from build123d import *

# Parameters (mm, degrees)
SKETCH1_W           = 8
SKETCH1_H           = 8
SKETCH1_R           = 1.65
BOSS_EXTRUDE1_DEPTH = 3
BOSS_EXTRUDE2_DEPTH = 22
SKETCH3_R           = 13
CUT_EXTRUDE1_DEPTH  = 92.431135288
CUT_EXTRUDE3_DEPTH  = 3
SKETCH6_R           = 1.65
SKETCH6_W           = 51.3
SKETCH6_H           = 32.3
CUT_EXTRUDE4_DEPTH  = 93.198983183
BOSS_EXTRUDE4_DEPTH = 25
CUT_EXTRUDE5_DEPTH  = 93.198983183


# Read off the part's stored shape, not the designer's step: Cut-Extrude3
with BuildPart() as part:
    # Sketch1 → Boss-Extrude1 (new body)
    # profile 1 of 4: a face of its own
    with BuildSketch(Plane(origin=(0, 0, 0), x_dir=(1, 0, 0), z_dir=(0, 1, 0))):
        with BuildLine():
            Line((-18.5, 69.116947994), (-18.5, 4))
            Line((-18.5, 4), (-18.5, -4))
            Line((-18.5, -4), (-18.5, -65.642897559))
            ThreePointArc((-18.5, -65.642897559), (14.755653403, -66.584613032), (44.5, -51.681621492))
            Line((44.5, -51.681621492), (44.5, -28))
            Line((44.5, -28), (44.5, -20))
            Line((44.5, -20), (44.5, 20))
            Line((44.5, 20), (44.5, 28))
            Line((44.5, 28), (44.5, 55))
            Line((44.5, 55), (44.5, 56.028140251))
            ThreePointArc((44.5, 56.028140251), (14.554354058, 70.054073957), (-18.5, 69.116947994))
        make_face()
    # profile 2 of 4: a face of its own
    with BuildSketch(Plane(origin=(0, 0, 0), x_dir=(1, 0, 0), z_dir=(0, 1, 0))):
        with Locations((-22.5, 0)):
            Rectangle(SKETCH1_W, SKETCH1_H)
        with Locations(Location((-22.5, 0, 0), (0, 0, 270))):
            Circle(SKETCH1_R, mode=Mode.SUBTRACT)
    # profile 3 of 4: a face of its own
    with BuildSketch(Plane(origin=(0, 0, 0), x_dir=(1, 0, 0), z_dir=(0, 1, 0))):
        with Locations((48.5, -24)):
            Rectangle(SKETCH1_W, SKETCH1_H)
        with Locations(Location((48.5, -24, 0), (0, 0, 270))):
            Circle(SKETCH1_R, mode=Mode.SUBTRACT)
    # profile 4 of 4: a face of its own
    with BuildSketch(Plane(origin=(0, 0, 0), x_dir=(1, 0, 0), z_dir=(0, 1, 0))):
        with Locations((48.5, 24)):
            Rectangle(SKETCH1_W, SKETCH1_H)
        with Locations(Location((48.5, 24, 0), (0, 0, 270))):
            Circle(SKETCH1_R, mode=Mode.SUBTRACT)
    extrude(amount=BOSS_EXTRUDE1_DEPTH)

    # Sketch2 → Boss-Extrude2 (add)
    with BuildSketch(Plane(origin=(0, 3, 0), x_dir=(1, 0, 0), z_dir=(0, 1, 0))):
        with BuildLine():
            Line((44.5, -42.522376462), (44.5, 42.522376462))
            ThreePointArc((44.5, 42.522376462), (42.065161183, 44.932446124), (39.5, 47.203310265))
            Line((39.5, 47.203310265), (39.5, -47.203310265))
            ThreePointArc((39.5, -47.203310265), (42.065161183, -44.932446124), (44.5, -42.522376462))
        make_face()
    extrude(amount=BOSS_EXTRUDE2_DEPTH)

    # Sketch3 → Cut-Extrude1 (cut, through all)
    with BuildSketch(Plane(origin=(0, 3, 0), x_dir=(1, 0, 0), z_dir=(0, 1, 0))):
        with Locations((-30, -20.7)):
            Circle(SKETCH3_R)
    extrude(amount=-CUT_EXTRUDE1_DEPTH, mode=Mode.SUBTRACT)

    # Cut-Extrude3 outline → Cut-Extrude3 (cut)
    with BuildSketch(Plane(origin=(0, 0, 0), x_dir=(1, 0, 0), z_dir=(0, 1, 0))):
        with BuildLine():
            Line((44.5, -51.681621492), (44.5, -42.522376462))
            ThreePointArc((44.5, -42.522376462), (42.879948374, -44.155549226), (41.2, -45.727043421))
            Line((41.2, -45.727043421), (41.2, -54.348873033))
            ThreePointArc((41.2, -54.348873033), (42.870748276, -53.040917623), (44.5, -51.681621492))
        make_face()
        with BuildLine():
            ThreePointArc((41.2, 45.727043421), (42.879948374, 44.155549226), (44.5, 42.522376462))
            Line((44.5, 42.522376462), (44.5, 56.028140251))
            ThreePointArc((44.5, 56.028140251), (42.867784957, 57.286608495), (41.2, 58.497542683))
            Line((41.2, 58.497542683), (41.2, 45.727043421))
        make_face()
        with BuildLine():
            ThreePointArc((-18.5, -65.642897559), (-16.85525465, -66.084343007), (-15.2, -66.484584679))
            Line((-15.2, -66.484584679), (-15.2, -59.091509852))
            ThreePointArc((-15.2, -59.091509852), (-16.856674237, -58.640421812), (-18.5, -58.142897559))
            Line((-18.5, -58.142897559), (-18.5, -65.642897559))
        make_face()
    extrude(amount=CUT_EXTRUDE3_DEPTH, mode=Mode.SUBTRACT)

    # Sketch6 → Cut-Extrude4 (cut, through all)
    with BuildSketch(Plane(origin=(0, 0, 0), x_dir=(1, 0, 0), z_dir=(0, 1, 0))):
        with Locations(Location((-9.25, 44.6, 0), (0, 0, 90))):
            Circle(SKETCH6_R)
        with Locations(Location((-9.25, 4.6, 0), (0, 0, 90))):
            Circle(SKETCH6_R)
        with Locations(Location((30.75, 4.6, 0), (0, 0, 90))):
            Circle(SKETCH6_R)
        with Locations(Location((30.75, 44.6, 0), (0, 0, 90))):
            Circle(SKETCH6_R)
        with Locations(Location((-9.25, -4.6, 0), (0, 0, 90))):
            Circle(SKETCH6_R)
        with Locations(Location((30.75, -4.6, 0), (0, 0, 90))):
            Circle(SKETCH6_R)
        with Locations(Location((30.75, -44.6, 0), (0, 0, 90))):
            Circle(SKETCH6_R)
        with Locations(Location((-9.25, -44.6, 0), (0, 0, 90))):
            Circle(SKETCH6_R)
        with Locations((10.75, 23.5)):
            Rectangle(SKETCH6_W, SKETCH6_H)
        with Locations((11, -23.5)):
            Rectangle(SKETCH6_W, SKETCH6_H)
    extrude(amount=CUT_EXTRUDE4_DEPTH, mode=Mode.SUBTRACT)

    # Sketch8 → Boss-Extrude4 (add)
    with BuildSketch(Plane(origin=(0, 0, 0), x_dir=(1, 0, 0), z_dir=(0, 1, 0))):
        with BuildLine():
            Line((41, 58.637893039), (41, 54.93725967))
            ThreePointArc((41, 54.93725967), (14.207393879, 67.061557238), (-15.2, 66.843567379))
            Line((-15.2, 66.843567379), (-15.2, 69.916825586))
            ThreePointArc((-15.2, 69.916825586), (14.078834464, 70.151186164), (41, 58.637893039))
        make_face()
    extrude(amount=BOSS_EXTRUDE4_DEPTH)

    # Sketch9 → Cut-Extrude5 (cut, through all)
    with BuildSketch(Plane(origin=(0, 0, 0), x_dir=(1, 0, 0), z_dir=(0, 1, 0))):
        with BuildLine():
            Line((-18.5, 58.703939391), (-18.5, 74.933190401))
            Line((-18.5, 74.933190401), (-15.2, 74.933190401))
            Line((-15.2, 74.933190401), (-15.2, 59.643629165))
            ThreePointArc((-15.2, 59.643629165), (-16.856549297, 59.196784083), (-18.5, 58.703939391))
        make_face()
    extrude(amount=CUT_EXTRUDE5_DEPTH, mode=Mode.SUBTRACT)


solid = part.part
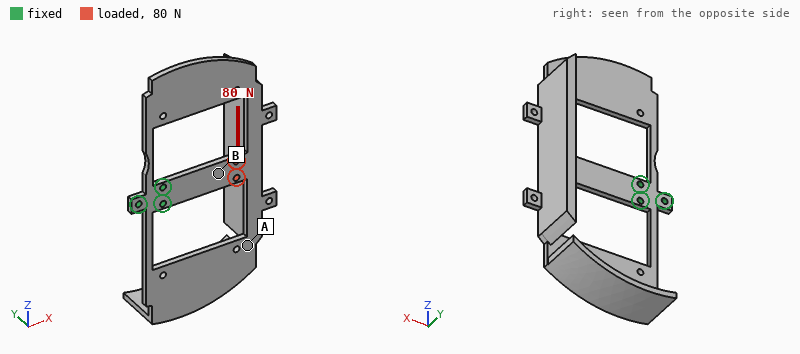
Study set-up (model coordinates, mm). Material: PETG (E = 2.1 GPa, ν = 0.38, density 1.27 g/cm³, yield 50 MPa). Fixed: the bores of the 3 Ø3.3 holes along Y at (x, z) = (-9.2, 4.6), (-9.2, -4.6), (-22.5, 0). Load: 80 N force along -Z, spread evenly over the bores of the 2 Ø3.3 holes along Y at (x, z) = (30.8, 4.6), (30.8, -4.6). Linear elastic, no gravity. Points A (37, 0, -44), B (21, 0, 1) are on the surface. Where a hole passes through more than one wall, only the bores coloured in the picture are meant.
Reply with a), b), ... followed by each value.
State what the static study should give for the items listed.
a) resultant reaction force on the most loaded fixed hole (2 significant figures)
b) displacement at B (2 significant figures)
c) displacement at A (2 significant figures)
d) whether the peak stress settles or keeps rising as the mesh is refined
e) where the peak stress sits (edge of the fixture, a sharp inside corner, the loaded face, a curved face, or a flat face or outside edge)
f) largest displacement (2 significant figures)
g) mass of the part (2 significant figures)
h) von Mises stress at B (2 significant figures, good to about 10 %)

a) 290 N
b) 0.62 mm
c) 1.6 mm
d) keeps rising
e) edge of the fixture
f) 1.9 mm
g) 36 g
h) 4.8 MPa
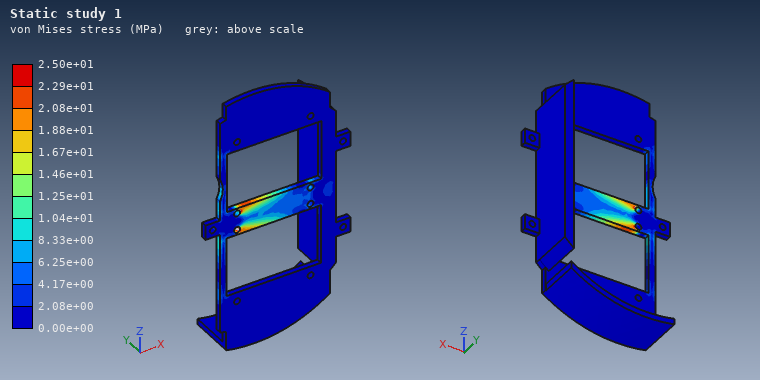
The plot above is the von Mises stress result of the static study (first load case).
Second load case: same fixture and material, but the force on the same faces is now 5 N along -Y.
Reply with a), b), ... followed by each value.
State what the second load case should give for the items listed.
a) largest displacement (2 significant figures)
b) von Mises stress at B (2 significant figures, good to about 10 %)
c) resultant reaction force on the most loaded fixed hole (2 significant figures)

a) 1.9 mm
b) 0.99 MPa
c) 3.8 N
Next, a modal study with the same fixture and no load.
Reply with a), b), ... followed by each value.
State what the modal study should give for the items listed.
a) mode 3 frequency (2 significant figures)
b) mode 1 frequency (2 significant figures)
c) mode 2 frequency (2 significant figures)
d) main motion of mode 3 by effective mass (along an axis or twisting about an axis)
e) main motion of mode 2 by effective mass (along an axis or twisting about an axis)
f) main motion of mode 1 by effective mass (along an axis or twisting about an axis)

a) 110 Hz
b) 39 Hz
c) 53 Hz
d) along Y
e) along Y
f) along Y
